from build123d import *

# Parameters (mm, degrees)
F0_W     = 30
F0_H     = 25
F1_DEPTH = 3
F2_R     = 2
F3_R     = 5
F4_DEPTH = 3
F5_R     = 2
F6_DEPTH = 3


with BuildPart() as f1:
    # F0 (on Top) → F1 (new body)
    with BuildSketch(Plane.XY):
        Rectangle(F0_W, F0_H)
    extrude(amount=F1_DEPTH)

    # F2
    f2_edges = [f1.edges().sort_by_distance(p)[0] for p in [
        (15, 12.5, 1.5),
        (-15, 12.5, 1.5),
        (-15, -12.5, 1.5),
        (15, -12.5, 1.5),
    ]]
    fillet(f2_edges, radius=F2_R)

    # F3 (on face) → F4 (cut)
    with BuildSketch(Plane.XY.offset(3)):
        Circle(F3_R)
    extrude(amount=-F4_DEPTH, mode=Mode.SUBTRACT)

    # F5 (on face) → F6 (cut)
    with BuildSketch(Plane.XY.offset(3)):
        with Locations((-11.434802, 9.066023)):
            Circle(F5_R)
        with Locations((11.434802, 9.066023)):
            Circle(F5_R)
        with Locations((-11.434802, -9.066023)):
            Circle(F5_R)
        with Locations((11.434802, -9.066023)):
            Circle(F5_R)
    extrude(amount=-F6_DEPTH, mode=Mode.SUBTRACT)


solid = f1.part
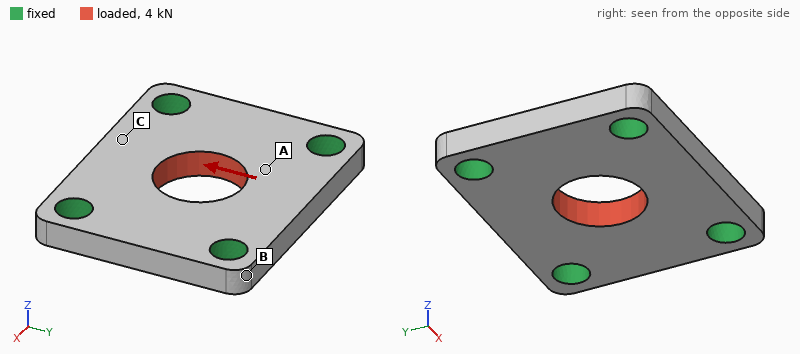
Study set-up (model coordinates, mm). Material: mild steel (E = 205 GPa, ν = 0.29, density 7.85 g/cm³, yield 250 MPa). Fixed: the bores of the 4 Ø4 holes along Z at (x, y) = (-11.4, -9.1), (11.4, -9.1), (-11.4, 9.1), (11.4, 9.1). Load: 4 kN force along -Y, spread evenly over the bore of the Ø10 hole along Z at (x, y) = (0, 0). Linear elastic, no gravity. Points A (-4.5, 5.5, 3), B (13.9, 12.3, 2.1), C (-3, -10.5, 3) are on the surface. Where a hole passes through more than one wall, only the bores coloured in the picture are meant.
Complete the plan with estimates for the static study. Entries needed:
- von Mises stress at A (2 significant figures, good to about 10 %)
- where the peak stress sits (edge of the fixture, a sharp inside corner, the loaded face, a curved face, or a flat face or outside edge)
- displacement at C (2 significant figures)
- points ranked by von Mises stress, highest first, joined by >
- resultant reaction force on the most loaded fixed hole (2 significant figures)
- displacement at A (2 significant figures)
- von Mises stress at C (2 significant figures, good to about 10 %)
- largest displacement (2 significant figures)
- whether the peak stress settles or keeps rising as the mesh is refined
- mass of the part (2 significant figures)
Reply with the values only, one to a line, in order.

44 MPa
edge of the fixture
2.9 µm
A > C > B
1.1 kN
2.6 µm
26 MPa
4.0 µm
keeps rising
15 g
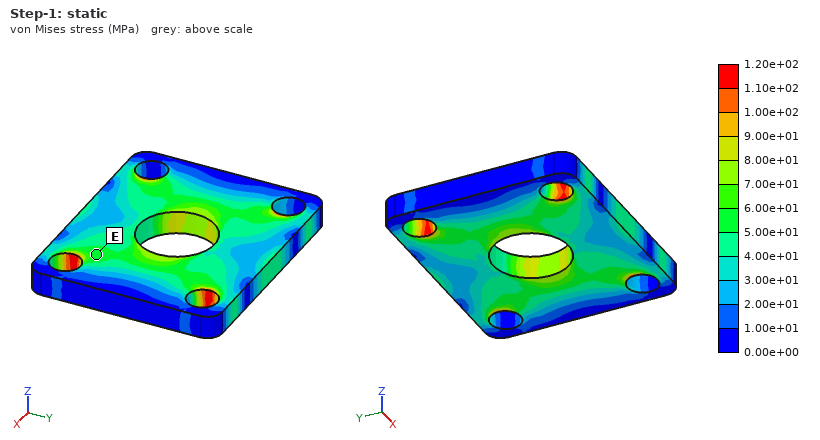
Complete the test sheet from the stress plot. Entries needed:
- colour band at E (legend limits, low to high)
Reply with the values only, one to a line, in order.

5.00e+01 to 6.00e+01 MPa
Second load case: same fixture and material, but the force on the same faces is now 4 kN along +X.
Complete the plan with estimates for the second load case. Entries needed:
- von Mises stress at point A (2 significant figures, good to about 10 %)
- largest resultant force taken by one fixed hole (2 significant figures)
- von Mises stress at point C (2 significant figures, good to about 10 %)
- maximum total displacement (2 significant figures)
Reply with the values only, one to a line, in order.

43 MPa
1.1 kN
13 MPa
2.5 µm
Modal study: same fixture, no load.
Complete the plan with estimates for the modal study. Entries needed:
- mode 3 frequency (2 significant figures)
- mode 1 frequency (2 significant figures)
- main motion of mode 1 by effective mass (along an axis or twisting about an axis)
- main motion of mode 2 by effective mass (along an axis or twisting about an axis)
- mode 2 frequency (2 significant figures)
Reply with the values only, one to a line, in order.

46 kHz
32 kHz
along Z
twisting about X
37 kHz
